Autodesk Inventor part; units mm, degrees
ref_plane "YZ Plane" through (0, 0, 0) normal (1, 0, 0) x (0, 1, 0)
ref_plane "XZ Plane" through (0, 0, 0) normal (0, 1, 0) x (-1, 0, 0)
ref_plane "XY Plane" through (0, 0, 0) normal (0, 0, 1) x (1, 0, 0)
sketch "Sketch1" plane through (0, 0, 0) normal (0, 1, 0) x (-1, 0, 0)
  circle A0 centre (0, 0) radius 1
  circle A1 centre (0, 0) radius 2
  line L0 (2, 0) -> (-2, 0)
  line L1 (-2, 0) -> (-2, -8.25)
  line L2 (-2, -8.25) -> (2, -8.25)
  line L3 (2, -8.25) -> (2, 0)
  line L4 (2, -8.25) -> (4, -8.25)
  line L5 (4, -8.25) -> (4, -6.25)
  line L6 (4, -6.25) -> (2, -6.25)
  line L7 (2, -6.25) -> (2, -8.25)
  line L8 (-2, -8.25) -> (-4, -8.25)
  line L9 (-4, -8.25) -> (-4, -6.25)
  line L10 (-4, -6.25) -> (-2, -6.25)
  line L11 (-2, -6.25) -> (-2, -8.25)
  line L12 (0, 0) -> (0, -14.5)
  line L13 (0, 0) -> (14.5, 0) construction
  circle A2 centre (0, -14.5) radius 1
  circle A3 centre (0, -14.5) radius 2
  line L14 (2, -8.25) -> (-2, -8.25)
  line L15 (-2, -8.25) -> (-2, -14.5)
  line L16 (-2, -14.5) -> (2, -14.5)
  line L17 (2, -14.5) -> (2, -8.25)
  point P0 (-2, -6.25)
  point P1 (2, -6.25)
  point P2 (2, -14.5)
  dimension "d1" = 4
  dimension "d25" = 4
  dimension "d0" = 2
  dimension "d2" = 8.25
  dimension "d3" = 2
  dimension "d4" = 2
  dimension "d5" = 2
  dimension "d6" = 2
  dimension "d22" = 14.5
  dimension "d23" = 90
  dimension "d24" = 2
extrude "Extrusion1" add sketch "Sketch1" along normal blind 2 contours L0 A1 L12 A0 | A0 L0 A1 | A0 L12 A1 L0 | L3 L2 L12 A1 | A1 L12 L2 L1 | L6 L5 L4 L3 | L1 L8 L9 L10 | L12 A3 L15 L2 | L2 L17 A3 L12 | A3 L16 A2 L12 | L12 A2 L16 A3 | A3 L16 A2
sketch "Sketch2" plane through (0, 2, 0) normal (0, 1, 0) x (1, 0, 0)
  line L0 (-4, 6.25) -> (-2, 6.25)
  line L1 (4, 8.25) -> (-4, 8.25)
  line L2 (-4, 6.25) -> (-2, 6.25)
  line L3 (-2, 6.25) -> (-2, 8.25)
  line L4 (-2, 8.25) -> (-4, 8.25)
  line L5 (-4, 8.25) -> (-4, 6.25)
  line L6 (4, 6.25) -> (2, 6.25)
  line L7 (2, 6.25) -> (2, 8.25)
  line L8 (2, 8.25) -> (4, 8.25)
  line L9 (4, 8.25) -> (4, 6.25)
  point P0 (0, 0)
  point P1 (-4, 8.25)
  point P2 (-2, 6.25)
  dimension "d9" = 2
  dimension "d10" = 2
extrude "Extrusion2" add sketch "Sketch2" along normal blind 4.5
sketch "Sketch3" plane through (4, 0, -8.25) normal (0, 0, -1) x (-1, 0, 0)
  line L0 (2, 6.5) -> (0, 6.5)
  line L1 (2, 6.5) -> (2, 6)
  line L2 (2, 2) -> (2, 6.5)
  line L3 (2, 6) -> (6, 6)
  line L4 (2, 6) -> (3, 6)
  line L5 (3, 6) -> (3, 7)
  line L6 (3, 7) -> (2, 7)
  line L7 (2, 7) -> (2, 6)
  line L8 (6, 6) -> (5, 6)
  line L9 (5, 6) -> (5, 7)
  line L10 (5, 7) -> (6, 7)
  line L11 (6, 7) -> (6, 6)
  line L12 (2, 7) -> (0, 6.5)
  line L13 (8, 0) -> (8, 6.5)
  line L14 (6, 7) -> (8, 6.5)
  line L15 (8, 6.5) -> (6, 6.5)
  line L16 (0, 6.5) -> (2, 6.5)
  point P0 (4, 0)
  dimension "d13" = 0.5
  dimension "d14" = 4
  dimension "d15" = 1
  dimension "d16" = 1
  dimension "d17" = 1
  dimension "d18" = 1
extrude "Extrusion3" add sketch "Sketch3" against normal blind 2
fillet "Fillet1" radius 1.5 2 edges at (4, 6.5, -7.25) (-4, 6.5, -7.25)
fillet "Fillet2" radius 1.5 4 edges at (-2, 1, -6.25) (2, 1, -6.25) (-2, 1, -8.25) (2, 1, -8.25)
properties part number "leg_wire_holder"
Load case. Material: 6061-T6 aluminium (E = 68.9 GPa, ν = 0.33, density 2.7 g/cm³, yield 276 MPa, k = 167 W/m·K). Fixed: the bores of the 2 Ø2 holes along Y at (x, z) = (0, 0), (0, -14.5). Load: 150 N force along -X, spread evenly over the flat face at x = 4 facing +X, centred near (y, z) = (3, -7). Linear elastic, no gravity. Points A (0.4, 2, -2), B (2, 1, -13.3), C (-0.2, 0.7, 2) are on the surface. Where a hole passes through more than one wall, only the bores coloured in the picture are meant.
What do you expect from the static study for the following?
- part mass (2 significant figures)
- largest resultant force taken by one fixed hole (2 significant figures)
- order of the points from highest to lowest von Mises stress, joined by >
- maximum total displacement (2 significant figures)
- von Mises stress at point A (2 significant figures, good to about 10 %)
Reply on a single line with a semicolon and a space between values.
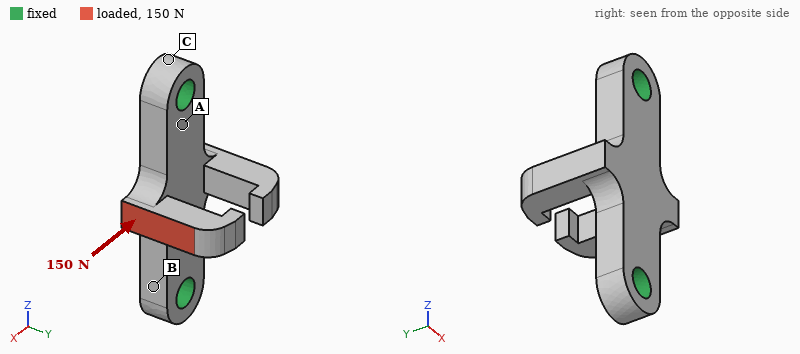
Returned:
0.51 g; 76 N; A > B > C; 61 µm; 71 MPa
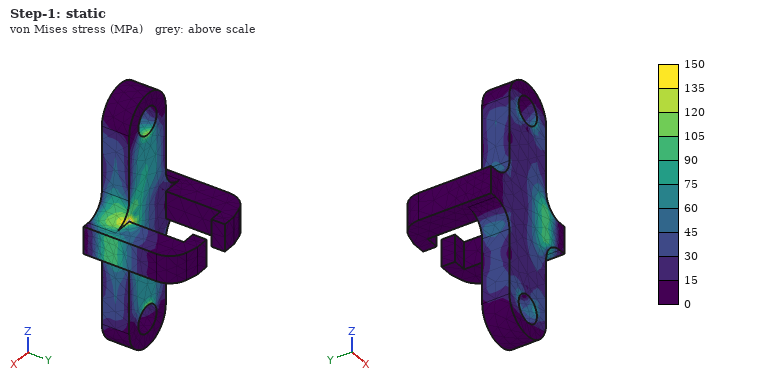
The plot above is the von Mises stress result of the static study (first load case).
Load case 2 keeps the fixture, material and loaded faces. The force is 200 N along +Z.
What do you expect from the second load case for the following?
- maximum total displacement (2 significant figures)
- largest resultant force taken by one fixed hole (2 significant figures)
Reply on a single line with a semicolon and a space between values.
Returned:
45 µm; 130 N
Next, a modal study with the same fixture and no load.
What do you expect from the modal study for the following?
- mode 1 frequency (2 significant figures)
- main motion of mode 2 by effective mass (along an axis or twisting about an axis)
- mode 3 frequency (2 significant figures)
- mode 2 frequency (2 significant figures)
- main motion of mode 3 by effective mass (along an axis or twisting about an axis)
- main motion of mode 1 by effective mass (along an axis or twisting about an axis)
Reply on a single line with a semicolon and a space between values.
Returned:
20 kHz; along Y; 34 kHz; 29 kHz; along Z; along X
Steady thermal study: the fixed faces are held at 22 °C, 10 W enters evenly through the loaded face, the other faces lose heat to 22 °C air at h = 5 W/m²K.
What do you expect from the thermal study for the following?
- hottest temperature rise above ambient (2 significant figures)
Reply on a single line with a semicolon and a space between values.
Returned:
61 K
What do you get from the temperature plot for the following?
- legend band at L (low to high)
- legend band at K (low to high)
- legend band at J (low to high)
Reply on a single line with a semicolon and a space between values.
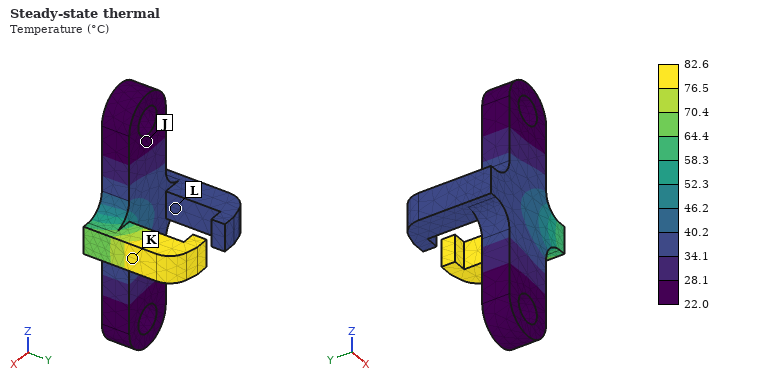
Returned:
34.1 to 40.2 °C; 76.5 to 82.6 °C; 22.0 to 28.1 °C
